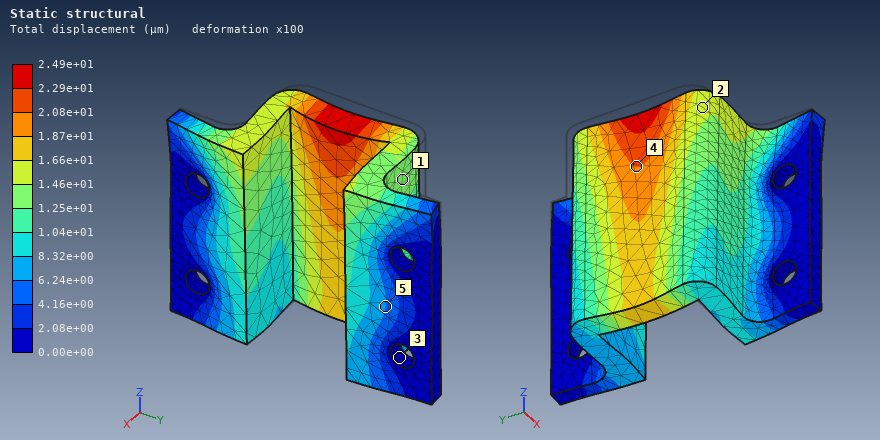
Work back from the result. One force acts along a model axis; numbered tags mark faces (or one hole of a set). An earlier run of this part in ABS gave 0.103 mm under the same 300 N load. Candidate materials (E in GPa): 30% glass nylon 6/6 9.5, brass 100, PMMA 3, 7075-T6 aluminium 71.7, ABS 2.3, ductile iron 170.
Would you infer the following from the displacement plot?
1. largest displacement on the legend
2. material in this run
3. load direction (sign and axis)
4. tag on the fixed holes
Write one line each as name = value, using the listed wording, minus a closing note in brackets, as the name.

largest displacement on the legend = 2.49e+01 µm
material in this run = 30% glass nylon 6/6
load direction = +X
tag on the fixed holes = 3
